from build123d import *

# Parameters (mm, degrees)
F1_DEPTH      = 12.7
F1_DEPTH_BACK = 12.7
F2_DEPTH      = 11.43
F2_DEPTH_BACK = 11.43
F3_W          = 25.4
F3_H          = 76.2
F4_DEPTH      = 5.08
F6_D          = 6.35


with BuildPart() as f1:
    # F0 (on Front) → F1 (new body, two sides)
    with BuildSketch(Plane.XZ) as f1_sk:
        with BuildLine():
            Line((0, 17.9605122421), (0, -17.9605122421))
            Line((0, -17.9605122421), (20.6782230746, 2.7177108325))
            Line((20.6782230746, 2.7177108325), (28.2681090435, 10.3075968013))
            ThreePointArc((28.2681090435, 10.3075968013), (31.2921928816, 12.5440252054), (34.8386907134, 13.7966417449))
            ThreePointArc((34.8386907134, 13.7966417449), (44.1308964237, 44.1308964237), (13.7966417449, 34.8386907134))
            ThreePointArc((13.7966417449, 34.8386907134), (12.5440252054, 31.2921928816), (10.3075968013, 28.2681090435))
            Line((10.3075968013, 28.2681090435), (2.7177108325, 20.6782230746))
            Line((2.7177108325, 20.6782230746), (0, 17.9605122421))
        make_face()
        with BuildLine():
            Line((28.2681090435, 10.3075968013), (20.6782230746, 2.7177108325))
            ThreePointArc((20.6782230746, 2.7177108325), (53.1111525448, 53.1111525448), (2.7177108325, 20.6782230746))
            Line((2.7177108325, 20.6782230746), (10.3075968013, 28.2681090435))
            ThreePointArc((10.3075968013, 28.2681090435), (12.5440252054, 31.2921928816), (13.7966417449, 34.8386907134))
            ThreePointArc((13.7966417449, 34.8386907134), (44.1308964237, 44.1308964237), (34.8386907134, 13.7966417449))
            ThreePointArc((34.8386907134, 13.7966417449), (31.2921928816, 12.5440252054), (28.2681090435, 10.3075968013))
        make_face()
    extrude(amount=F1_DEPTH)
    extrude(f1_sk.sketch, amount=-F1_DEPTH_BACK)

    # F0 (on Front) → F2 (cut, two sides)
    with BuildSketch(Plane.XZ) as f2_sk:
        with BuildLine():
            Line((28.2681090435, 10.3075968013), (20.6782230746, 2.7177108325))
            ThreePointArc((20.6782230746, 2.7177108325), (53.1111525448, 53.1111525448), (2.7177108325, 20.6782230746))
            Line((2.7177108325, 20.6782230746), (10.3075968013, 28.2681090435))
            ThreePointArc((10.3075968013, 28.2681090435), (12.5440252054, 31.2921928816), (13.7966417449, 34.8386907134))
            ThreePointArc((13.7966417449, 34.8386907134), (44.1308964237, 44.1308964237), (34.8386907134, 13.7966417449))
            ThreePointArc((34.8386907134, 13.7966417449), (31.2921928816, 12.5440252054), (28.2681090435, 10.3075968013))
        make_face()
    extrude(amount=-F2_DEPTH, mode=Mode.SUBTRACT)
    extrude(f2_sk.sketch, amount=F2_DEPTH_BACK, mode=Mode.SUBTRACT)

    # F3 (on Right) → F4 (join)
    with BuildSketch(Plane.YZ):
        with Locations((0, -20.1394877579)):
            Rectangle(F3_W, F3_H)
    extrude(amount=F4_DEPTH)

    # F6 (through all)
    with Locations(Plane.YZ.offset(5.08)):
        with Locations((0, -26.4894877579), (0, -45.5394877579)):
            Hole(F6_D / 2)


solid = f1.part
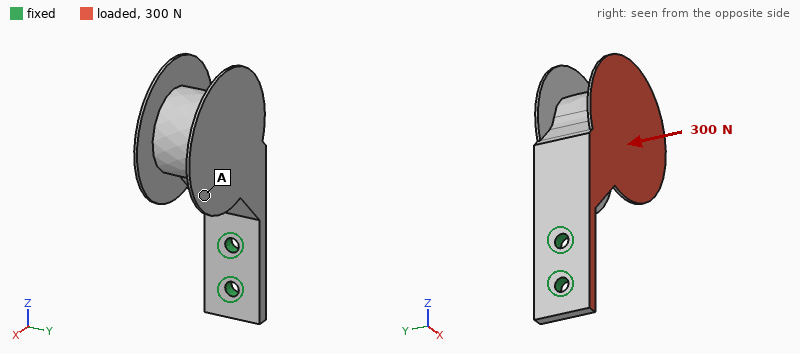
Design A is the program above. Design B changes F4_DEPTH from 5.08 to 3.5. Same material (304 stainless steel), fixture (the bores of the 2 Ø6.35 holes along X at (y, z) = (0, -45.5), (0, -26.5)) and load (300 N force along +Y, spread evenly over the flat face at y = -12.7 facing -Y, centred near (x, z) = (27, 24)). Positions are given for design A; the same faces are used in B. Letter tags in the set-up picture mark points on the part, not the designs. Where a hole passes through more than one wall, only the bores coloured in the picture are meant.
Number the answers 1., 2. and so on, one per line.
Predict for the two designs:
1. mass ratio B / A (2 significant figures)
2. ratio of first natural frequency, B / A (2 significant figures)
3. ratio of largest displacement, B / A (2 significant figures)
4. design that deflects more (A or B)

1. 0.97
2. 0.62
3. 2.0
4. B
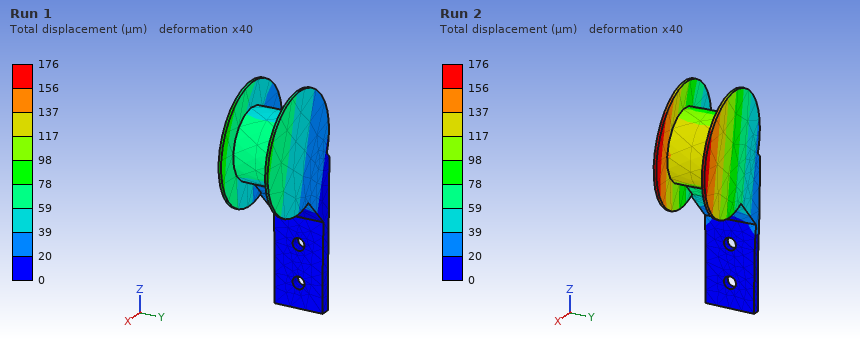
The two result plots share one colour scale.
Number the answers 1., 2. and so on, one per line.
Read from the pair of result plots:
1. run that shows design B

1. Run 2
